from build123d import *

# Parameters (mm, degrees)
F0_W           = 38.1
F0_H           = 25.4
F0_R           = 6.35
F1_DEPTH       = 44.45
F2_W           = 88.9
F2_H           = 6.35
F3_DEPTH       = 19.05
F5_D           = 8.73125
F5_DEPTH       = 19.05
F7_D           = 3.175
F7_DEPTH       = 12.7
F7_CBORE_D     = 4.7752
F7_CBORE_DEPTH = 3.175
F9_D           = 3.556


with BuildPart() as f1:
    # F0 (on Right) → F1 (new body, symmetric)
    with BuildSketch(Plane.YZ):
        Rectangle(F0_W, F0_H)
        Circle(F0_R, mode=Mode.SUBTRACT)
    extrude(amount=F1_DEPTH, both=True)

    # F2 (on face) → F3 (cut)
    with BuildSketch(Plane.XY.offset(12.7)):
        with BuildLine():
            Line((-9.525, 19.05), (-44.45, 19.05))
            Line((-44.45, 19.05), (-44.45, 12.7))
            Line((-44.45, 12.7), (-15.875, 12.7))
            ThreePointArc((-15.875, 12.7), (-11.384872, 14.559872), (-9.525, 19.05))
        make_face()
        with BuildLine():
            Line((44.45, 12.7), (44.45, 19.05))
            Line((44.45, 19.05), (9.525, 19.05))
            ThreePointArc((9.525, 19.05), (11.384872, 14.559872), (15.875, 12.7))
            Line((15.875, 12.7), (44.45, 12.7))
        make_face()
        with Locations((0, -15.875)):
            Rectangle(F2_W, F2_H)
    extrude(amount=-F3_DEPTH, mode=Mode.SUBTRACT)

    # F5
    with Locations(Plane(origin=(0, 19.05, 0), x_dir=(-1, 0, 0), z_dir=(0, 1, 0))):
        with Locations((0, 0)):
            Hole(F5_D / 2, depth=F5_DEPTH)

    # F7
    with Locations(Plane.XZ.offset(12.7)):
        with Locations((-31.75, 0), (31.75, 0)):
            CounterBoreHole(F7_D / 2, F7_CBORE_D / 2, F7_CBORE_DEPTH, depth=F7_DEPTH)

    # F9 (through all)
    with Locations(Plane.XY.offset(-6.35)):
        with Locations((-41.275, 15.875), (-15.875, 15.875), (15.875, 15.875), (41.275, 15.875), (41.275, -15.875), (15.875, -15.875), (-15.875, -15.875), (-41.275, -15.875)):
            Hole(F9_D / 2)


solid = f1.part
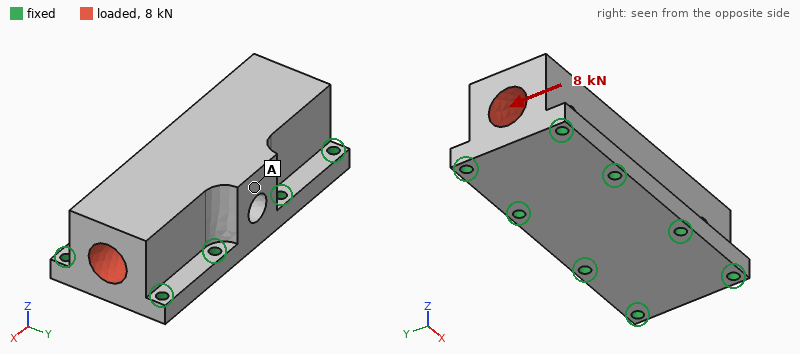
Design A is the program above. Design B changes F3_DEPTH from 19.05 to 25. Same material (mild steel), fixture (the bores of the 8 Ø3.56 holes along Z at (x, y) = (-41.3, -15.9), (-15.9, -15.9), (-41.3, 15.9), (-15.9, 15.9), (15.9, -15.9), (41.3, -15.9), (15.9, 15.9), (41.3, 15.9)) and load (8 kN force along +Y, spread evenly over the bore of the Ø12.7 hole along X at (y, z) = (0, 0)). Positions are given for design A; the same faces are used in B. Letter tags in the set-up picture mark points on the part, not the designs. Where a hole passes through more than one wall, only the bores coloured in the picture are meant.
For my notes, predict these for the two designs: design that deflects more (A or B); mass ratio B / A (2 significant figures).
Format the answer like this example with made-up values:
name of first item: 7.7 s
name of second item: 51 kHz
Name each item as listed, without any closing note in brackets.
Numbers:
design that deflects more: B
mass ratio B / A: 0.90
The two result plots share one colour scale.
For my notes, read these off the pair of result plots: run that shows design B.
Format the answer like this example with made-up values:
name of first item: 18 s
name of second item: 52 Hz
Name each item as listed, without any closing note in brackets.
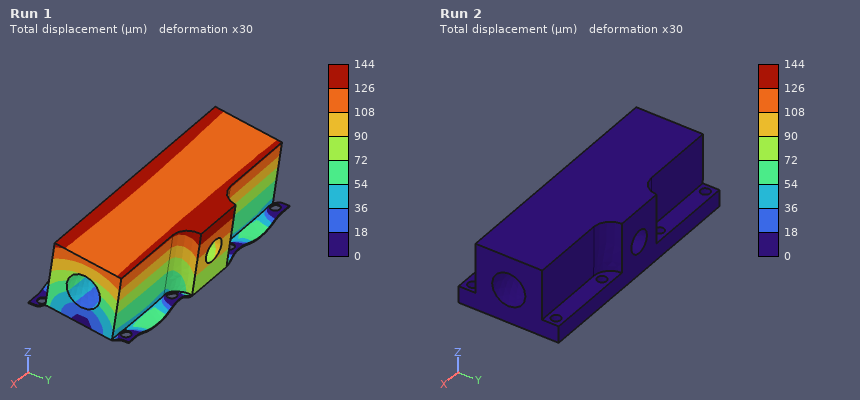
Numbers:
run that shows design B: Run 1
